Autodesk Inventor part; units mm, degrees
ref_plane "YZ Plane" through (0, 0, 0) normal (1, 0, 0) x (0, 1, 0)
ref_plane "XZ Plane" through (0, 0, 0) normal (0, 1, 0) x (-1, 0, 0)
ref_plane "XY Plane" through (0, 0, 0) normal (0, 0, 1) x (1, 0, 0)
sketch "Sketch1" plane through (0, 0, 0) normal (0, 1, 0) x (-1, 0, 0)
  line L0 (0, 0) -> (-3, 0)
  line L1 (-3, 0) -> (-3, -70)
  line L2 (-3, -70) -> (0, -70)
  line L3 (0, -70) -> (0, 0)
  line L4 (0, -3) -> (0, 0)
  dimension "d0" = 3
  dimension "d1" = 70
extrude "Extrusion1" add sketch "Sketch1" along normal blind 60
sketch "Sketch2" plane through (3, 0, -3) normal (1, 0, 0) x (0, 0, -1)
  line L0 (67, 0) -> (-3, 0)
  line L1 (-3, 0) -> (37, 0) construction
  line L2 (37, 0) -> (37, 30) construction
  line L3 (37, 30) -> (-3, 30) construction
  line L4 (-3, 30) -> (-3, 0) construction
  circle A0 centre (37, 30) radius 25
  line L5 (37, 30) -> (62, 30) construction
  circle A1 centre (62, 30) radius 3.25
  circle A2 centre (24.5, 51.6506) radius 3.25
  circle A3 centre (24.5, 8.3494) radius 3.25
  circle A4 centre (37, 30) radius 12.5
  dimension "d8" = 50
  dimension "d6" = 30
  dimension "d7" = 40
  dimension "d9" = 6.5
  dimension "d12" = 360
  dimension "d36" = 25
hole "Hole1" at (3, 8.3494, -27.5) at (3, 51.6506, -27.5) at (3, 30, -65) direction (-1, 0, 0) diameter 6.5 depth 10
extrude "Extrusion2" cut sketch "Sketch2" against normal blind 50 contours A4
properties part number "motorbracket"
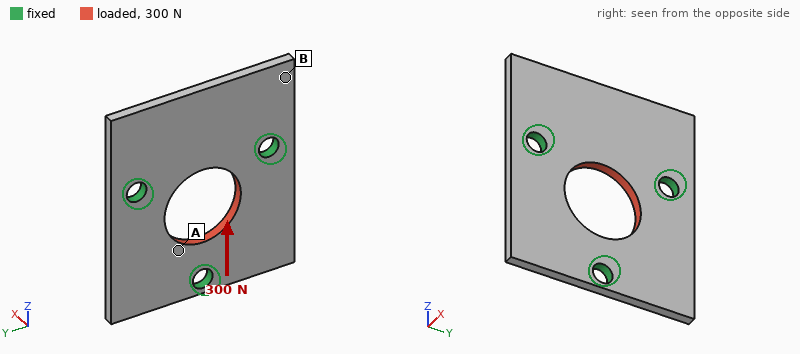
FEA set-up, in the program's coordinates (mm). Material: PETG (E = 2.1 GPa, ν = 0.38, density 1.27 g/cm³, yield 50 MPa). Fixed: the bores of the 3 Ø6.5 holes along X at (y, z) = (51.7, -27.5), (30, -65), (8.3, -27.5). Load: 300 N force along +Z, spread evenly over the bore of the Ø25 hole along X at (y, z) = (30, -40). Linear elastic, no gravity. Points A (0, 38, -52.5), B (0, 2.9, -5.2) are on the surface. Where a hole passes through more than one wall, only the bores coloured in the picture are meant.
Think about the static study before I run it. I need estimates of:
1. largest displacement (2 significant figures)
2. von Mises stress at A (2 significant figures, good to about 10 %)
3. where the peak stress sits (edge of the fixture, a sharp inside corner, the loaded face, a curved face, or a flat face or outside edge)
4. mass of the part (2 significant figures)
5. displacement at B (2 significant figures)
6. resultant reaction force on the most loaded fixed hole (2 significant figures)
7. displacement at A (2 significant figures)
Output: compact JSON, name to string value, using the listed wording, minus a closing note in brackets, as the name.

{"largest displacement": "23 µm", "von Mises stress at A": "1.6 MPa", "where the peak stress sits": "edge of the fixture", "mass of the part": "14 g", "displacement at B": "5.3 µm", "resultant reaction force on the most loaded fixed hole": "110 N", "displacement at A": "13 µm"}
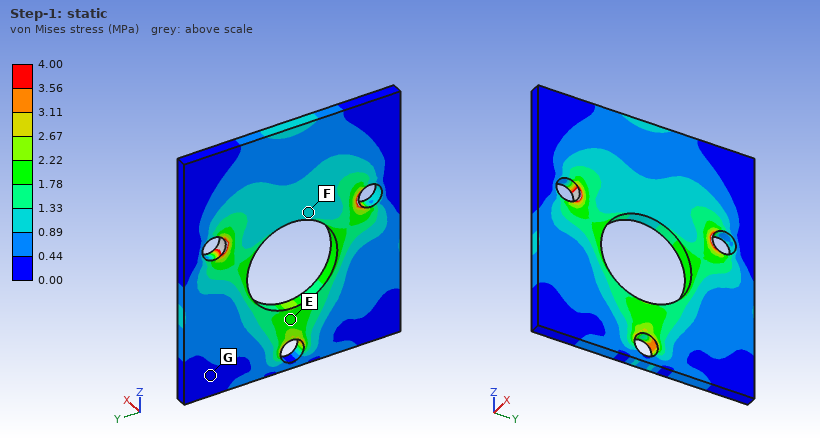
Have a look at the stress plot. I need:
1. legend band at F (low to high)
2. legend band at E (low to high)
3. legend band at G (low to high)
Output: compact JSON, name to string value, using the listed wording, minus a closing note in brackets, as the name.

{"legend band at F": "0.89 to 1.33 MPa", "legend band at E": "1.78 to 2.22 MPa", "legend band at G": "0.00 to 0.44 MPa"}
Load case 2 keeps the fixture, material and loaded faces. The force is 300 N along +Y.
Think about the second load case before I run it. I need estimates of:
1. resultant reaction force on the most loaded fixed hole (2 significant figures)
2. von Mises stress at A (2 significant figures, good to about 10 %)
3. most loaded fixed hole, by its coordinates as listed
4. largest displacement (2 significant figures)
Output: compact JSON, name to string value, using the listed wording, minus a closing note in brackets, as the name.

{"resultant reaction force on the most loaded fixed hole": "110 N", "von Mises stress at A": "1.3 MPa", "most loaded fixed hole, by its coordinates as listed": "(30, -65)", "largest displacement": "25 µm"}
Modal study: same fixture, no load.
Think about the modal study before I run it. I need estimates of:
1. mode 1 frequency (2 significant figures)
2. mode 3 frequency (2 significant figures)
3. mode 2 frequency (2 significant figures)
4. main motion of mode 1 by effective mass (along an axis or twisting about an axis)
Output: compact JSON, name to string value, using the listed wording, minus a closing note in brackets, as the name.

{"mode 1 frequency": "810 Hz", "mode 3 frequency": "1100 Hz", "mode 2 frequency": "1100 Hz", "main motion of mode 1 by effective mass": "along X"}
